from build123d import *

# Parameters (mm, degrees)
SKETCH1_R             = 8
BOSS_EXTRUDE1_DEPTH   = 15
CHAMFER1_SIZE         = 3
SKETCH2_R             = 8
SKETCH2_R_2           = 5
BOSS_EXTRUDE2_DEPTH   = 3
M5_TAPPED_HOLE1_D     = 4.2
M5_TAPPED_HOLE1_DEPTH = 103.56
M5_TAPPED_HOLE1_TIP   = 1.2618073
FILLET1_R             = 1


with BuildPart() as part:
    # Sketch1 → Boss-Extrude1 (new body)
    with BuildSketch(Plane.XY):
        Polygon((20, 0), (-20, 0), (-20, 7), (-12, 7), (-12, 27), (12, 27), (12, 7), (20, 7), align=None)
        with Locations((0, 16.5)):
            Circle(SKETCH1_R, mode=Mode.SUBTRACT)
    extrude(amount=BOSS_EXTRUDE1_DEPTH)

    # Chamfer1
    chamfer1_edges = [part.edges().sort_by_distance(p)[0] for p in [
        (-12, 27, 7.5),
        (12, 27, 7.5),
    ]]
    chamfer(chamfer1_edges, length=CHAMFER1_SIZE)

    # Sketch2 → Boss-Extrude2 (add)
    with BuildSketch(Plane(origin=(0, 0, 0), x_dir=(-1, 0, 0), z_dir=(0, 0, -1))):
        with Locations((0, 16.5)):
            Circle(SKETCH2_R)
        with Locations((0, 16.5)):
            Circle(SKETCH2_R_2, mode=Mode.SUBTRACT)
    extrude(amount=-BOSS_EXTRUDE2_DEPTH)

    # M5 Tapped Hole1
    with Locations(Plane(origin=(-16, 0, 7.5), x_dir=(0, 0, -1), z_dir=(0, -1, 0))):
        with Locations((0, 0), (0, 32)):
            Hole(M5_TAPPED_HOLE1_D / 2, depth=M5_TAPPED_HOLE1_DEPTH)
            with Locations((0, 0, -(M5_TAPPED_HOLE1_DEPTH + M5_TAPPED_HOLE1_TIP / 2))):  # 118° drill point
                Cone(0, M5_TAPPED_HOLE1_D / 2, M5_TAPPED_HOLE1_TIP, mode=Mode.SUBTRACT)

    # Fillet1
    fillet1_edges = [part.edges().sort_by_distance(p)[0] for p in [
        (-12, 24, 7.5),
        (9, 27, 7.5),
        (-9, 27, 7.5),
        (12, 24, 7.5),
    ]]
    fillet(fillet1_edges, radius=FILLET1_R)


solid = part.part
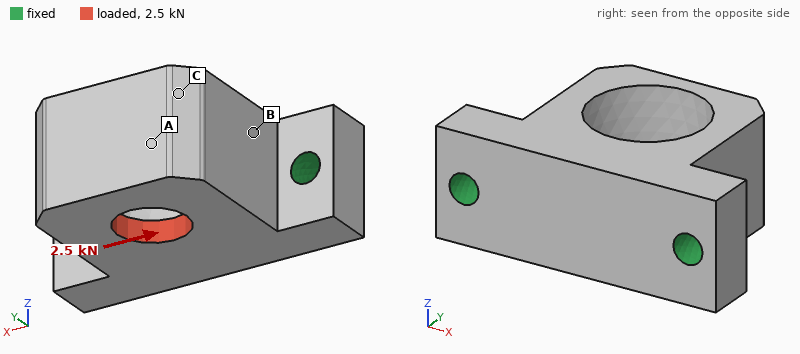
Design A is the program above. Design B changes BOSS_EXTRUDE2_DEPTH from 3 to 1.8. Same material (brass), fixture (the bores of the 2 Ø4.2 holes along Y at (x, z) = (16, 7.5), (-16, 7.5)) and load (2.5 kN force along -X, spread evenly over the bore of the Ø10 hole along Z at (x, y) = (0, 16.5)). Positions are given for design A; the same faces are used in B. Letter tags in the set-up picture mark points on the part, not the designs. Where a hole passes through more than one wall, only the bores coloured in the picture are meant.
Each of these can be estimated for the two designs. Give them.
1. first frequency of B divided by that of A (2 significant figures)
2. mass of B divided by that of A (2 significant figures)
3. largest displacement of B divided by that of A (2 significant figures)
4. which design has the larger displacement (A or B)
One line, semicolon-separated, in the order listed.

1.0; 0.98; 1.2; B
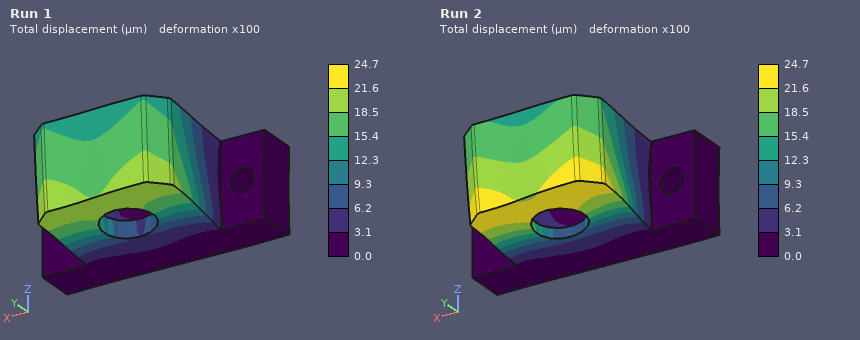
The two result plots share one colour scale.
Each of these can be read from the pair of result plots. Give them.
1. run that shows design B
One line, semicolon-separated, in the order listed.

Run 2
